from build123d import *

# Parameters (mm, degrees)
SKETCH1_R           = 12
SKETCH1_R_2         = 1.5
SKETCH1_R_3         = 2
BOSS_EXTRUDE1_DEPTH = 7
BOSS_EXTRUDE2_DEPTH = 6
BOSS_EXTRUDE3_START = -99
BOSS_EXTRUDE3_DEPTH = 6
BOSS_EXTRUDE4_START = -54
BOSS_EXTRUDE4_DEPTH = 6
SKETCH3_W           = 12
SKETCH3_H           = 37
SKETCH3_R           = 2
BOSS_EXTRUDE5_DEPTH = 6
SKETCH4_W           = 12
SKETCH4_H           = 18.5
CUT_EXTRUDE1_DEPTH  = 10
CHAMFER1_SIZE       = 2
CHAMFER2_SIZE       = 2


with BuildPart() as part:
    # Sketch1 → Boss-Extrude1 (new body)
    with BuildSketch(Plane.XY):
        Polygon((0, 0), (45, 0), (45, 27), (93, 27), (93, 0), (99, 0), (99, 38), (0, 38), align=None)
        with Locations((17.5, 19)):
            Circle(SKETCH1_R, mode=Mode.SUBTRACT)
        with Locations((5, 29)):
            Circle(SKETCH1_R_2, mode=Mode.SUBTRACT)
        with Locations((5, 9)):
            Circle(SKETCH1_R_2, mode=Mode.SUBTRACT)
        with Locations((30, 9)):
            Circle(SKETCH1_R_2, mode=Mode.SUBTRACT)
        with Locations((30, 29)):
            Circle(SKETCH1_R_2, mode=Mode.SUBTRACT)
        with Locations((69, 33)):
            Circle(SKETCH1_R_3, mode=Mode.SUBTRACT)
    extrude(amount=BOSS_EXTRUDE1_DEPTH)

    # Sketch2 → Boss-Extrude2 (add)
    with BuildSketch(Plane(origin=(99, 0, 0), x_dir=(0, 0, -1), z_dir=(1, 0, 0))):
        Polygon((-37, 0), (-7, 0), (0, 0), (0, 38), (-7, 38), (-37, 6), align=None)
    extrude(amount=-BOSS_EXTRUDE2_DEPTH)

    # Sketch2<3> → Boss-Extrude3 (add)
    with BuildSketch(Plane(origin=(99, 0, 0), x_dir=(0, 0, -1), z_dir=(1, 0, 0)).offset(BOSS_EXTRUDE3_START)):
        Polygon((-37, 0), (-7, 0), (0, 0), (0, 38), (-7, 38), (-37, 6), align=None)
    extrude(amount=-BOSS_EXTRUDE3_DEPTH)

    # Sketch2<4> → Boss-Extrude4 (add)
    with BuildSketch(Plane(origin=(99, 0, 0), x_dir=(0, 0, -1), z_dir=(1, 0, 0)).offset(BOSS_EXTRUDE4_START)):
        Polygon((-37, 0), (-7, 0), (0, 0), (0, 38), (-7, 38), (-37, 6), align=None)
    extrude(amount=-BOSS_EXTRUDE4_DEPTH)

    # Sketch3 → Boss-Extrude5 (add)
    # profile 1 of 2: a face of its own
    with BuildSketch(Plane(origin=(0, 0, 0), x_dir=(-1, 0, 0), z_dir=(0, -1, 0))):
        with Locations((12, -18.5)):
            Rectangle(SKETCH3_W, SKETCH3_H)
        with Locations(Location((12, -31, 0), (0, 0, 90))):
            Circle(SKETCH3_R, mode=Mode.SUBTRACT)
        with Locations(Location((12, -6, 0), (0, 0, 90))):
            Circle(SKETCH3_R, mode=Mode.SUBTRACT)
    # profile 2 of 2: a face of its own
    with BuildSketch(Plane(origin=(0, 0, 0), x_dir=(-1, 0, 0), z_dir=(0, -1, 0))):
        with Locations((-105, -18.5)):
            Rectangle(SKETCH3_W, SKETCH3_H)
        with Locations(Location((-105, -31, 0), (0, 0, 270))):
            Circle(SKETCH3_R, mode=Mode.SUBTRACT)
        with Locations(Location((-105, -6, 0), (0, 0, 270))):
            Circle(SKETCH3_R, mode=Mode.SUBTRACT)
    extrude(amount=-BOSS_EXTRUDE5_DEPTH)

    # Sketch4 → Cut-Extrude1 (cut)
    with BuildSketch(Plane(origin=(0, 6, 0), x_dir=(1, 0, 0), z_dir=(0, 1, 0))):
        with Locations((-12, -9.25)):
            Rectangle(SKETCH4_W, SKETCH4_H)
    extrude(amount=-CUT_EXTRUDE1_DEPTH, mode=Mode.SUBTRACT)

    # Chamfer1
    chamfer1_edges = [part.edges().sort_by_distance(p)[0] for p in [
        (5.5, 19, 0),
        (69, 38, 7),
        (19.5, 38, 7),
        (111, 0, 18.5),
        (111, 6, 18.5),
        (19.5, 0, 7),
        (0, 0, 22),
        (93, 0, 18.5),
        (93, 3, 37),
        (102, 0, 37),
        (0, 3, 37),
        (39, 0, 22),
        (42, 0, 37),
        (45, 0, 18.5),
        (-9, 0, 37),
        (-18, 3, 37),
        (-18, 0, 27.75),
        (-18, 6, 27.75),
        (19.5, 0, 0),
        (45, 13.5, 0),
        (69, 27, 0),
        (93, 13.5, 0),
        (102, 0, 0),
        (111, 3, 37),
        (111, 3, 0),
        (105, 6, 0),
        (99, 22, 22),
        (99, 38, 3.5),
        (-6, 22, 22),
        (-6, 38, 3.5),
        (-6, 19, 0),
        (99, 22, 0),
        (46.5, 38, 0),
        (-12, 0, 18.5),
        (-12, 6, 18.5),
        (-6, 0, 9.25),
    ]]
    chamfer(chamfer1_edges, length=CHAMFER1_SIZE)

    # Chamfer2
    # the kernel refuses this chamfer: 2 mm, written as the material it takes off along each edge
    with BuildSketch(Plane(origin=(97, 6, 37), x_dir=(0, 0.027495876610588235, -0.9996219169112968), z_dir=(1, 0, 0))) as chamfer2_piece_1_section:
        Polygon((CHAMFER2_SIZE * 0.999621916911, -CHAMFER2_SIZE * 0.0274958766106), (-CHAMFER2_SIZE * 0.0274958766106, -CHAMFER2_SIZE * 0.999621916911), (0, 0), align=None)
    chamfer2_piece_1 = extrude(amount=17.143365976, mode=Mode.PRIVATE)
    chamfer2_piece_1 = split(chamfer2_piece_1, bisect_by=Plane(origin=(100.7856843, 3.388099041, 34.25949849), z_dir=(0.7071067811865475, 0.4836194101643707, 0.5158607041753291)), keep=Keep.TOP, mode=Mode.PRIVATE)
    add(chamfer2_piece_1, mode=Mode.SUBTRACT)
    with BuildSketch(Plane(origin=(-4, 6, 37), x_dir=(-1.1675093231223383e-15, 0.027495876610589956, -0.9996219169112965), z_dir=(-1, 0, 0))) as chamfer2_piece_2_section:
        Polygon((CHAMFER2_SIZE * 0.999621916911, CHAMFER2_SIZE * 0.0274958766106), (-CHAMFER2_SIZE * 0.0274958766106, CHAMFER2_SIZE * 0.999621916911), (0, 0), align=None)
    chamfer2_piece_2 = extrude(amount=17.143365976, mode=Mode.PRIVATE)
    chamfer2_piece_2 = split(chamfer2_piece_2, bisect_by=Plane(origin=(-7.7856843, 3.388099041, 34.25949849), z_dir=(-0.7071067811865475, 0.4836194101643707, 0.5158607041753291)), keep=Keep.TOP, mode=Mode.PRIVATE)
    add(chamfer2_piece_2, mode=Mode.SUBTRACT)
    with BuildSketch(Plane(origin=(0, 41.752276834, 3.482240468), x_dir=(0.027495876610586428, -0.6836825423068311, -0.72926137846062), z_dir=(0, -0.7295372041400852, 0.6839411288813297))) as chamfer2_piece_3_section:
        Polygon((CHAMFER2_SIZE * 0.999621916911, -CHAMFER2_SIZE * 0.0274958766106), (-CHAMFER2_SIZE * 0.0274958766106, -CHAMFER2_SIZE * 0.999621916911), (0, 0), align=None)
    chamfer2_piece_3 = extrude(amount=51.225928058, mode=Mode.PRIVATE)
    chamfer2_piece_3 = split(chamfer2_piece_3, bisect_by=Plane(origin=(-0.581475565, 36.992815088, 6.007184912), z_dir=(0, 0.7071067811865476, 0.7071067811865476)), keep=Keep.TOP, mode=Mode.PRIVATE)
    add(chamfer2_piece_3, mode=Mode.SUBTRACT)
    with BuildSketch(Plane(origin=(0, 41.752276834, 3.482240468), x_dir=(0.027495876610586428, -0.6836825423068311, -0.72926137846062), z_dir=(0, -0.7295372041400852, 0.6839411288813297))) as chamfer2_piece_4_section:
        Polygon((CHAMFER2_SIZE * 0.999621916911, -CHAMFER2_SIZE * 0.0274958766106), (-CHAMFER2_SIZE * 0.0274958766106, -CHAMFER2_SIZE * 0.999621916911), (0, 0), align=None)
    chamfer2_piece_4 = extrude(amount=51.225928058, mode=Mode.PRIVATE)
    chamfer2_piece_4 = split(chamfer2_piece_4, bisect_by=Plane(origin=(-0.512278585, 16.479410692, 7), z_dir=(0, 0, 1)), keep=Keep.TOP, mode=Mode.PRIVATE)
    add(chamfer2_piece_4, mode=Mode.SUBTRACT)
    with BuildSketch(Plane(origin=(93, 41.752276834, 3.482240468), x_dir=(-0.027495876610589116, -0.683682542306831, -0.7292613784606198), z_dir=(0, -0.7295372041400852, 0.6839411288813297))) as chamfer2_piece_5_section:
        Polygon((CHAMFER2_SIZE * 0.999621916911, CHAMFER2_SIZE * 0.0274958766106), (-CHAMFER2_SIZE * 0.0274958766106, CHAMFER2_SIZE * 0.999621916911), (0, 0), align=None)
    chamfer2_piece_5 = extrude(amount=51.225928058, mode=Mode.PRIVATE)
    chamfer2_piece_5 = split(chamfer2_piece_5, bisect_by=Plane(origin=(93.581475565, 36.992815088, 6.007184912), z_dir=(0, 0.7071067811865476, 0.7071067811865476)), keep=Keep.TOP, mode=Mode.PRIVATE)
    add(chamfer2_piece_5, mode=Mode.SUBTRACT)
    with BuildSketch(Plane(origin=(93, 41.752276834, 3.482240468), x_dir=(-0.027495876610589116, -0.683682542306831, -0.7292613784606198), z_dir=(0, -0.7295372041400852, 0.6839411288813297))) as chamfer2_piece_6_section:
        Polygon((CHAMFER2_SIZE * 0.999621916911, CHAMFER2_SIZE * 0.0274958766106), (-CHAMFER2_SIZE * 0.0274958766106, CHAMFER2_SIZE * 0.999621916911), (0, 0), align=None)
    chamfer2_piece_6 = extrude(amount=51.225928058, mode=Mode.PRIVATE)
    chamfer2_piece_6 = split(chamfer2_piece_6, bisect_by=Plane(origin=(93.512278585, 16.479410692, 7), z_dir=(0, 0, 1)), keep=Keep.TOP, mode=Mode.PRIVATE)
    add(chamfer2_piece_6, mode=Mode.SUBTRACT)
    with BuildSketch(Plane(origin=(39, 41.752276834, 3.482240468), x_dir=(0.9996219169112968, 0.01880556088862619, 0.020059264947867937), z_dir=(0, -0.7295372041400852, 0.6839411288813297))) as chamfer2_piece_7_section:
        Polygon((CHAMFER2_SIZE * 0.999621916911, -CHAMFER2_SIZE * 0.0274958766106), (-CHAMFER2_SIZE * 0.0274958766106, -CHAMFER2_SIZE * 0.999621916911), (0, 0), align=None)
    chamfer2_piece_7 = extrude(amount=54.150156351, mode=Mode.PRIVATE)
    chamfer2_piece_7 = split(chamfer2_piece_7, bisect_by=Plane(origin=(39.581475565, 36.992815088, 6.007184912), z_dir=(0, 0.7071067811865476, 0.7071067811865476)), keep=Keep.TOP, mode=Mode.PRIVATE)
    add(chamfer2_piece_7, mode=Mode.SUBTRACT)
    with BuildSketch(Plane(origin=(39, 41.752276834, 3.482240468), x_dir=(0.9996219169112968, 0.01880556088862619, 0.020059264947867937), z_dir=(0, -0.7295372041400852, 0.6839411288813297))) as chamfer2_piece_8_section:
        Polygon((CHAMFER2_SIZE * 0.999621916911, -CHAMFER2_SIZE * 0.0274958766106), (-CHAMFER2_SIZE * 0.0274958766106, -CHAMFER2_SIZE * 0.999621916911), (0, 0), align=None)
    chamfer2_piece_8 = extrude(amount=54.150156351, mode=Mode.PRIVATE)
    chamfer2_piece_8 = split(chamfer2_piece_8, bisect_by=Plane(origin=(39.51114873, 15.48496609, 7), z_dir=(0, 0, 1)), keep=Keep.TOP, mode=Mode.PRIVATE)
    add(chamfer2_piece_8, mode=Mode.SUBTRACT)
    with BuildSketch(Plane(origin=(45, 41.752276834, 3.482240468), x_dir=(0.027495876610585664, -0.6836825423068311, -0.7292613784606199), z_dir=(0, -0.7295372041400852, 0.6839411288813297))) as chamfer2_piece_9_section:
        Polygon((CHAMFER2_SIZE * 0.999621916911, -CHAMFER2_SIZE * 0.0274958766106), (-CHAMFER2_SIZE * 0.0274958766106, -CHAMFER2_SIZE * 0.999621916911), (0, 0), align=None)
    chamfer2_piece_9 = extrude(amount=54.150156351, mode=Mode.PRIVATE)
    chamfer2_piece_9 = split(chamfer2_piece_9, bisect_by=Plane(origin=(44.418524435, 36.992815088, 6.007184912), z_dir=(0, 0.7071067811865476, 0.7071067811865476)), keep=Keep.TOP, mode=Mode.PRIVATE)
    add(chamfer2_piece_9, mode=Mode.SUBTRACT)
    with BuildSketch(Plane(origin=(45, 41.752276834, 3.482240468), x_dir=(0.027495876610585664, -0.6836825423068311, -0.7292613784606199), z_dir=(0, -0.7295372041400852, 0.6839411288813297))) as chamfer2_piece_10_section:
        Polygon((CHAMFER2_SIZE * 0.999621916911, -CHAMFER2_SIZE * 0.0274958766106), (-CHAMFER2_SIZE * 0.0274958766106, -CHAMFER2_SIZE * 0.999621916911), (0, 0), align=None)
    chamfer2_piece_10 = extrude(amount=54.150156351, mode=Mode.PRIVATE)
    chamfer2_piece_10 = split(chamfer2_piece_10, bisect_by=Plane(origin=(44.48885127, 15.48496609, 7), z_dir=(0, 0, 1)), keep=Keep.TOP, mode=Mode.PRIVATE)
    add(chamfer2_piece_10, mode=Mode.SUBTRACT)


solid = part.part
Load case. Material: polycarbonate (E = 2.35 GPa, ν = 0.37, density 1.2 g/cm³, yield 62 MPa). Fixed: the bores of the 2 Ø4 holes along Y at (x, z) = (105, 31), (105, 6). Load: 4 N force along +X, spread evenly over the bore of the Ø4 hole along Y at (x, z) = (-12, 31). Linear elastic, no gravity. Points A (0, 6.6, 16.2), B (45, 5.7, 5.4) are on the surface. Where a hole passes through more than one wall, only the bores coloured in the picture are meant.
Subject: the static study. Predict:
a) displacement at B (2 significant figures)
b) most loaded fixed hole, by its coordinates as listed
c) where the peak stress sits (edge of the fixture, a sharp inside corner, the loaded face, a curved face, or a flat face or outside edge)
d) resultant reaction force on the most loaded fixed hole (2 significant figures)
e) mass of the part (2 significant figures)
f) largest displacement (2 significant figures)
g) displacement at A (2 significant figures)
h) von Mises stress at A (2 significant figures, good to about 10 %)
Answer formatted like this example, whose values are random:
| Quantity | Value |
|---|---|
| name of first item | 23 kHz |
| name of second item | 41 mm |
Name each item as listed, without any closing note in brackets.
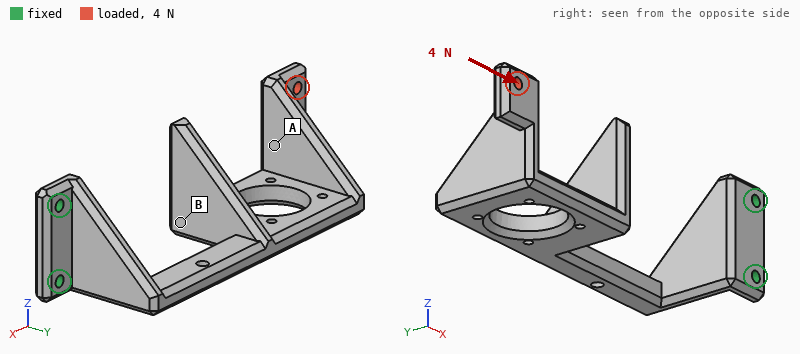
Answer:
| Quantity | Value |
|---|---|
| displacement at B | 0.45 mm |
| most loaded fixed hole, by its coordinates as listed | (105, 31) |
| where the peak stress sits | a curved face |
| resultant reaction force on the most loaded fixed hole | 4.1 N |
| mass of the part | 34 g |
| largest displacement | 1.6 mm |
| displacement at A | 1.2 mm |
| von Mises stress at A | 0.54 MPa |
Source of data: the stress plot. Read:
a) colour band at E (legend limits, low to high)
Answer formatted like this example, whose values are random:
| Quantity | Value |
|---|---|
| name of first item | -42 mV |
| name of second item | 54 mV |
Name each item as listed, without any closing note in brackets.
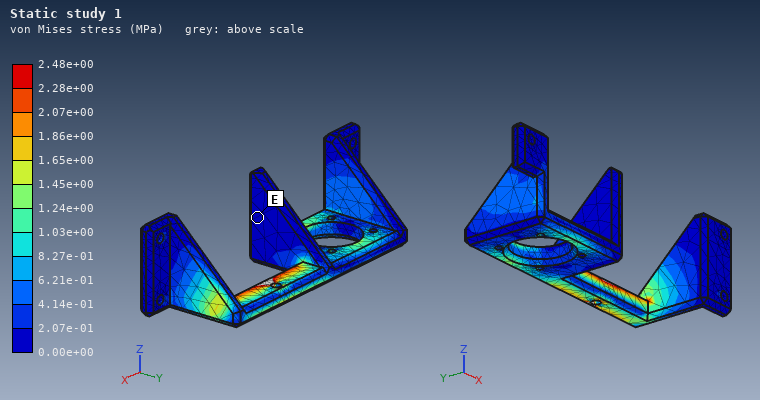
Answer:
| Quantity | Value |
|---|---|
| colour band at E | 0.00e+00 to 2.07e-01 MPa |
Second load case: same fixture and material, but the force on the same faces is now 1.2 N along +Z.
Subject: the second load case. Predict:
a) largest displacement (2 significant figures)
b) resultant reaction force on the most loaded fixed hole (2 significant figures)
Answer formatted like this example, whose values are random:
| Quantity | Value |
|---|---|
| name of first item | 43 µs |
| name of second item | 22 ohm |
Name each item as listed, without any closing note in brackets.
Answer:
| Quantity | Value |
|---|---|
| largest displacement | 1.5 mm |
| resultant reaction force on the most loaded fixed hole | 5.8 N |
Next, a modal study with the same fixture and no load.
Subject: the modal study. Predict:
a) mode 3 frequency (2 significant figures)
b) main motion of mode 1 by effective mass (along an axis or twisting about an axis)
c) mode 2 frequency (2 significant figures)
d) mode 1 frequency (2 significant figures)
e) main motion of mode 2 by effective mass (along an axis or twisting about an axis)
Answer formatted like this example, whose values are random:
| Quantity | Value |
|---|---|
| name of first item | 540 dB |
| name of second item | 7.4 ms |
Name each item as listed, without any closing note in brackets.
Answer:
| Quantity | Value |
|---|---|
| mode 3 frequency | 220 Hz |
| main motion of mode 1 by effective mass | along Z |
| mode 2 frequency | 53 Hz |
| mode 1 frequency | 47 Hz |
| main motion of mode 2 by effective mass | along Y |
